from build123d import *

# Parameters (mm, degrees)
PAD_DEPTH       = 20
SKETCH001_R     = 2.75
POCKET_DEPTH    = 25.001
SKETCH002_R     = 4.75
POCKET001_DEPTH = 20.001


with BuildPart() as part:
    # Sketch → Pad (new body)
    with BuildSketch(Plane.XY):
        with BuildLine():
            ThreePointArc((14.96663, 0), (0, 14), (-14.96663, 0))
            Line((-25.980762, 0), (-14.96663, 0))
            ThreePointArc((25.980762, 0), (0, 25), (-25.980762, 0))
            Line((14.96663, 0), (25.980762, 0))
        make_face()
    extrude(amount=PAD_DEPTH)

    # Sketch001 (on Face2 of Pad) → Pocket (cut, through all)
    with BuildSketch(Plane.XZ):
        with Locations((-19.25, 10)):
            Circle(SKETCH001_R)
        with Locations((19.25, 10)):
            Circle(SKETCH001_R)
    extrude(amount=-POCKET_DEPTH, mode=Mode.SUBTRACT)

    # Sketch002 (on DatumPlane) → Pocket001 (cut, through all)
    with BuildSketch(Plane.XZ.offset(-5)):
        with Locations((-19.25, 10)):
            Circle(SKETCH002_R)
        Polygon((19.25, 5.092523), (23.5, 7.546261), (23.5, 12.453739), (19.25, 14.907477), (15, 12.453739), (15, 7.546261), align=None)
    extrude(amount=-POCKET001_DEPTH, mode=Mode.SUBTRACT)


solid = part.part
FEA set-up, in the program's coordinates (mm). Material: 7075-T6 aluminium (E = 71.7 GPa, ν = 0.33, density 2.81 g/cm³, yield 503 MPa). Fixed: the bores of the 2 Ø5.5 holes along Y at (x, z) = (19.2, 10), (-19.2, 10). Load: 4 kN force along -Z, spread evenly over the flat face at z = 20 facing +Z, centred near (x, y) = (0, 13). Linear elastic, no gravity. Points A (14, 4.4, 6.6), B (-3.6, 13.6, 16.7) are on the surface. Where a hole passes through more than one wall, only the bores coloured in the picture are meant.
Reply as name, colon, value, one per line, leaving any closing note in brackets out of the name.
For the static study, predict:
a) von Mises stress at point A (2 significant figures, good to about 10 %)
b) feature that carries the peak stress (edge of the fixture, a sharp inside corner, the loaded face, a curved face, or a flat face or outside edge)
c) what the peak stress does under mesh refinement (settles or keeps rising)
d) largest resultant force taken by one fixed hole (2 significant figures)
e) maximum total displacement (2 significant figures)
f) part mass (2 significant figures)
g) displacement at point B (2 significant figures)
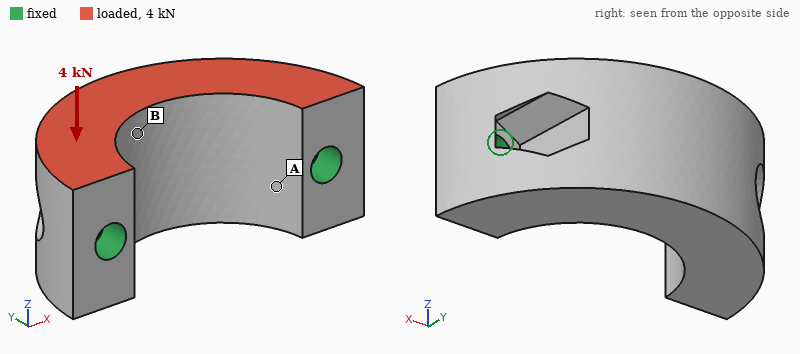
von Mises stress at point A: 68 MPa
feature that carries the peak stress: edge of the fixture
what the peak stress does under mesh refinement: keeps rising
largest resultant force taken by one fixed hole: 2.0 kN
maximum total displacement: 77 µm
part mass: 34 g
displacement at point B: 44 µm
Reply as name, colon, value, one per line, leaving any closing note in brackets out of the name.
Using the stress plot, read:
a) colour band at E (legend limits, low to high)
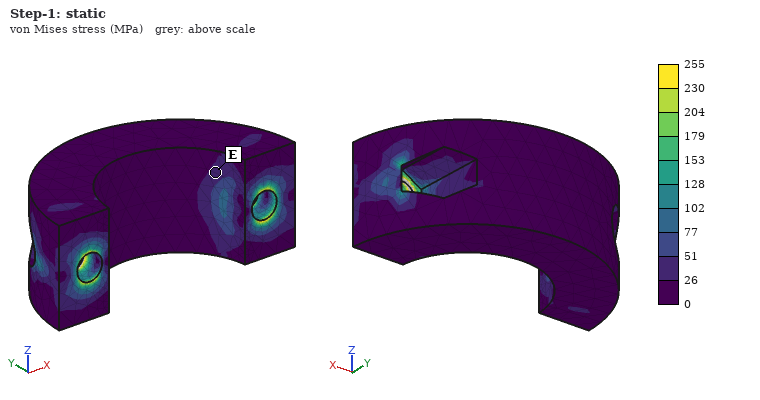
colour band at E: 26 to 51 MPa
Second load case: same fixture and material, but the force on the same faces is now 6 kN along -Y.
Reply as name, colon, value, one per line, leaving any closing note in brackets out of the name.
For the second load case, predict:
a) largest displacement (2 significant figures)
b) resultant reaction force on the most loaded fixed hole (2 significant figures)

largest displacement: 0.10 mm
resultant reaction force on the most loaded fixed hole: 3.1 kN
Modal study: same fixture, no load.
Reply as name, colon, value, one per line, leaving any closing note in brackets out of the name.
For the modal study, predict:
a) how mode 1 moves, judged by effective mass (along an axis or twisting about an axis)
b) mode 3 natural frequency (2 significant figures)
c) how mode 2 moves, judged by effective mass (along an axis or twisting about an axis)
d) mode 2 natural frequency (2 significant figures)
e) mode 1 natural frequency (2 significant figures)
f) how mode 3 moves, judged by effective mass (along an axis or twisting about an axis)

how mode 1 moves, judged by effective mass: along Z
mode 3 natural frequency: 19 kHz
how mode 2 moves, judged by effective mass: along X
mode 2 natural frequency: 16 kHz
mode 1 natural frequency: 7200 Hz
how mode 3 moves, judged by effective mass: twisting about Y
